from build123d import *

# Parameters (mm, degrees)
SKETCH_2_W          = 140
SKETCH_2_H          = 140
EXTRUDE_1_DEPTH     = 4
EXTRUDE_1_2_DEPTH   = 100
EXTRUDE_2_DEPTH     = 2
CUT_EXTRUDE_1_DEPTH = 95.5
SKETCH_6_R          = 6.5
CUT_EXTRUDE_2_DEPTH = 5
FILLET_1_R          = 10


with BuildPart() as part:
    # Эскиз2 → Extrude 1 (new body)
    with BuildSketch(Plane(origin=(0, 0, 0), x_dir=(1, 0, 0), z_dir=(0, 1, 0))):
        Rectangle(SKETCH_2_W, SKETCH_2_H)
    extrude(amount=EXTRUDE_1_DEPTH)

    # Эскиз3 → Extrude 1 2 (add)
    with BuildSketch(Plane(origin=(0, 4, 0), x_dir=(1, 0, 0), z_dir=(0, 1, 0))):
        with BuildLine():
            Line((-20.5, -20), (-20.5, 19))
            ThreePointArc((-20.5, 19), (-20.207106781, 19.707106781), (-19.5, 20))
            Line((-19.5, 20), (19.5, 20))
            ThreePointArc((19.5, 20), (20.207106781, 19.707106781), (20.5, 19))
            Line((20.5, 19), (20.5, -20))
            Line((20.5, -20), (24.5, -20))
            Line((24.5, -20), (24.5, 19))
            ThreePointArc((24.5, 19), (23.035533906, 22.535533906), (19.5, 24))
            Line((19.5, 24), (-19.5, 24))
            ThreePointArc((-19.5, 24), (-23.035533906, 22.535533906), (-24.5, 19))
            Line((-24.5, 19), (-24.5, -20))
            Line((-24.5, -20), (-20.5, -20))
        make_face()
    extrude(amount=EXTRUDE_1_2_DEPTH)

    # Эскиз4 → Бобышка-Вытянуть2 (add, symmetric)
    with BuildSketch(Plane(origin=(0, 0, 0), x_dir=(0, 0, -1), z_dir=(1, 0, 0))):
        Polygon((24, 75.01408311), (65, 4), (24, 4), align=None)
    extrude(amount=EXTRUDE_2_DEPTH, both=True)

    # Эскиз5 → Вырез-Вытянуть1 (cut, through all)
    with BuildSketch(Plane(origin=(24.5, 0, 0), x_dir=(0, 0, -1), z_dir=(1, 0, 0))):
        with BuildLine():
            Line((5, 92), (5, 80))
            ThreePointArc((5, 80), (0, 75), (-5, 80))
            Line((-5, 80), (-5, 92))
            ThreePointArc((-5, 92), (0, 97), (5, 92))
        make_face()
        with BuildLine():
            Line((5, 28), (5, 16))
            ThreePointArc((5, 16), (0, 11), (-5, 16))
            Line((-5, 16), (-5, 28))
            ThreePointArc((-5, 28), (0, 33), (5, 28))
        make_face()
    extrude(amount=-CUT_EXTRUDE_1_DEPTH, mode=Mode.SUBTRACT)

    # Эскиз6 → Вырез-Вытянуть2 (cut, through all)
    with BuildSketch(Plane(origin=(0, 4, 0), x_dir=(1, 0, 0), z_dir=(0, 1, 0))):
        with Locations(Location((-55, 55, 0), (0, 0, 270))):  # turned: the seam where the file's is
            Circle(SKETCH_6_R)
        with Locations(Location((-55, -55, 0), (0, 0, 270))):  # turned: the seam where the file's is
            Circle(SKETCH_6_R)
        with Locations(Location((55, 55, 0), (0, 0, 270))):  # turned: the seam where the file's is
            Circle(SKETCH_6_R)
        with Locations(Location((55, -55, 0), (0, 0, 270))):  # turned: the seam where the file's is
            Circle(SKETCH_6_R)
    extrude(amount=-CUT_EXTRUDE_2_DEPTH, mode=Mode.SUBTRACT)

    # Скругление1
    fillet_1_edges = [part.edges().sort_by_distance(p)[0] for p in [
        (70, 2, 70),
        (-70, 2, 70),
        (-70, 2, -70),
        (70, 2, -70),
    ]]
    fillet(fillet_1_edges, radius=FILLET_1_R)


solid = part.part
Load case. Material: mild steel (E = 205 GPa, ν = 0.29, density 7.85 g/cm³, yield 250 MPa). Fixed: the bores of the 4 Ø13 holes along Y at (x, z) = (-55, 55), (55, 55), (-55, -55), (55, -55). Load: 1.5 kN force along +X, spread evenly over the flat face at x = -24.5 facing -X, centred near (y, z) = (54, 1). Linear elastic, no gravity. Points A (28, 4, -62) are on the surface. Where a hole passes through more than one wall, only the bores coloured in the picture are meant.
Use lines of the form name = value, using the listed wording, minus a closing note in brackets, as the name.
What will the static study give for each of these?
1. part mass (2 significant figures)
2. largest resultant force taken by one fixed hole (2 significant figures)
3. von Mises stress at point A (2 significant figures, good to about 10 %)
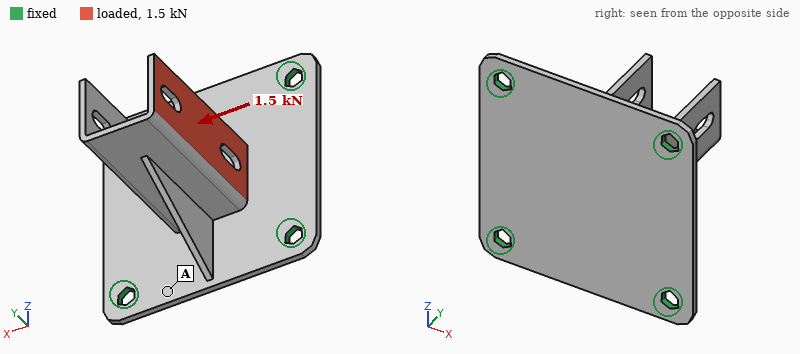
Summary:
part mass = 1.0 kg
largest resultant force taken by one fixed hole = 800 N
von Mises stress at point A = 17 MPa
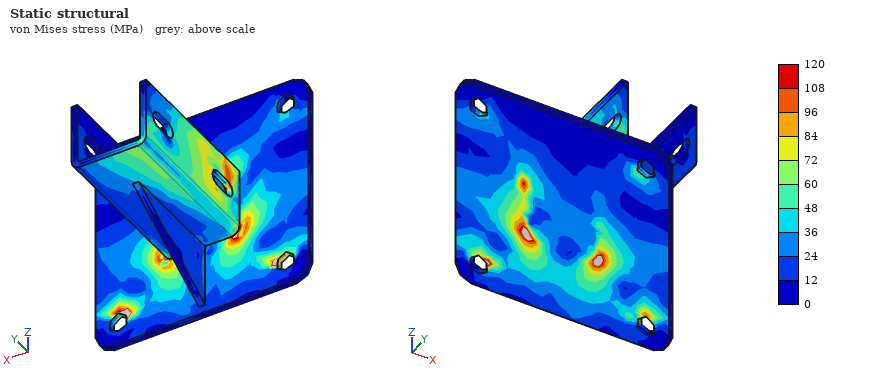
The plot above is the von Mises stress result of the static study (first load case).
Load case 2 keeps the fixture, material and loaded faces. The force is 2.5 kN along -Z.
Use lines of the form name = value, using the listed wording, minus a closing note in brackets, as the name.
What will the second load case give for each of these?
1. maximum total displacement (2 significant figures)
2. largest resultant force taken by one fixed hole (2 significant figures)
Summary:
maximum total displacement = 0.53 mm
largest resultant force taken by one fixed hole = 1.2 kN
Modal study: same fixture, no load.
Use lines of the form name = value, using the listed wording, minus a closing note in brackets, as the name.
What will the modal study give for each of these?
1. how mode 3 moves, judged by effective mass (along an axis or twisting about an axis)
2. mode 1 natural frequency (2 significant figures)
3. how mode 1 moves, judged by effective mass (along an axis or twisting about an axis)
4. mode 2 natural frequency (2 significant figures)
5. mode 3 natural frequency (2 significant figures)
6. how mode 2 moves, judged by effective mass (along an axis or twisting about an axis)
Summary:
how mode 3 moves, judged by effective mass = along Y
mode 1 natural frequency = 640 Hz
how mode 1 moves, judged by effective mass = along X
mode 2 natural frequency = 850 Hz
mode 3 natural frequency = 1000 Hz
how mode 2 moves, judged by effective mass = along Z
